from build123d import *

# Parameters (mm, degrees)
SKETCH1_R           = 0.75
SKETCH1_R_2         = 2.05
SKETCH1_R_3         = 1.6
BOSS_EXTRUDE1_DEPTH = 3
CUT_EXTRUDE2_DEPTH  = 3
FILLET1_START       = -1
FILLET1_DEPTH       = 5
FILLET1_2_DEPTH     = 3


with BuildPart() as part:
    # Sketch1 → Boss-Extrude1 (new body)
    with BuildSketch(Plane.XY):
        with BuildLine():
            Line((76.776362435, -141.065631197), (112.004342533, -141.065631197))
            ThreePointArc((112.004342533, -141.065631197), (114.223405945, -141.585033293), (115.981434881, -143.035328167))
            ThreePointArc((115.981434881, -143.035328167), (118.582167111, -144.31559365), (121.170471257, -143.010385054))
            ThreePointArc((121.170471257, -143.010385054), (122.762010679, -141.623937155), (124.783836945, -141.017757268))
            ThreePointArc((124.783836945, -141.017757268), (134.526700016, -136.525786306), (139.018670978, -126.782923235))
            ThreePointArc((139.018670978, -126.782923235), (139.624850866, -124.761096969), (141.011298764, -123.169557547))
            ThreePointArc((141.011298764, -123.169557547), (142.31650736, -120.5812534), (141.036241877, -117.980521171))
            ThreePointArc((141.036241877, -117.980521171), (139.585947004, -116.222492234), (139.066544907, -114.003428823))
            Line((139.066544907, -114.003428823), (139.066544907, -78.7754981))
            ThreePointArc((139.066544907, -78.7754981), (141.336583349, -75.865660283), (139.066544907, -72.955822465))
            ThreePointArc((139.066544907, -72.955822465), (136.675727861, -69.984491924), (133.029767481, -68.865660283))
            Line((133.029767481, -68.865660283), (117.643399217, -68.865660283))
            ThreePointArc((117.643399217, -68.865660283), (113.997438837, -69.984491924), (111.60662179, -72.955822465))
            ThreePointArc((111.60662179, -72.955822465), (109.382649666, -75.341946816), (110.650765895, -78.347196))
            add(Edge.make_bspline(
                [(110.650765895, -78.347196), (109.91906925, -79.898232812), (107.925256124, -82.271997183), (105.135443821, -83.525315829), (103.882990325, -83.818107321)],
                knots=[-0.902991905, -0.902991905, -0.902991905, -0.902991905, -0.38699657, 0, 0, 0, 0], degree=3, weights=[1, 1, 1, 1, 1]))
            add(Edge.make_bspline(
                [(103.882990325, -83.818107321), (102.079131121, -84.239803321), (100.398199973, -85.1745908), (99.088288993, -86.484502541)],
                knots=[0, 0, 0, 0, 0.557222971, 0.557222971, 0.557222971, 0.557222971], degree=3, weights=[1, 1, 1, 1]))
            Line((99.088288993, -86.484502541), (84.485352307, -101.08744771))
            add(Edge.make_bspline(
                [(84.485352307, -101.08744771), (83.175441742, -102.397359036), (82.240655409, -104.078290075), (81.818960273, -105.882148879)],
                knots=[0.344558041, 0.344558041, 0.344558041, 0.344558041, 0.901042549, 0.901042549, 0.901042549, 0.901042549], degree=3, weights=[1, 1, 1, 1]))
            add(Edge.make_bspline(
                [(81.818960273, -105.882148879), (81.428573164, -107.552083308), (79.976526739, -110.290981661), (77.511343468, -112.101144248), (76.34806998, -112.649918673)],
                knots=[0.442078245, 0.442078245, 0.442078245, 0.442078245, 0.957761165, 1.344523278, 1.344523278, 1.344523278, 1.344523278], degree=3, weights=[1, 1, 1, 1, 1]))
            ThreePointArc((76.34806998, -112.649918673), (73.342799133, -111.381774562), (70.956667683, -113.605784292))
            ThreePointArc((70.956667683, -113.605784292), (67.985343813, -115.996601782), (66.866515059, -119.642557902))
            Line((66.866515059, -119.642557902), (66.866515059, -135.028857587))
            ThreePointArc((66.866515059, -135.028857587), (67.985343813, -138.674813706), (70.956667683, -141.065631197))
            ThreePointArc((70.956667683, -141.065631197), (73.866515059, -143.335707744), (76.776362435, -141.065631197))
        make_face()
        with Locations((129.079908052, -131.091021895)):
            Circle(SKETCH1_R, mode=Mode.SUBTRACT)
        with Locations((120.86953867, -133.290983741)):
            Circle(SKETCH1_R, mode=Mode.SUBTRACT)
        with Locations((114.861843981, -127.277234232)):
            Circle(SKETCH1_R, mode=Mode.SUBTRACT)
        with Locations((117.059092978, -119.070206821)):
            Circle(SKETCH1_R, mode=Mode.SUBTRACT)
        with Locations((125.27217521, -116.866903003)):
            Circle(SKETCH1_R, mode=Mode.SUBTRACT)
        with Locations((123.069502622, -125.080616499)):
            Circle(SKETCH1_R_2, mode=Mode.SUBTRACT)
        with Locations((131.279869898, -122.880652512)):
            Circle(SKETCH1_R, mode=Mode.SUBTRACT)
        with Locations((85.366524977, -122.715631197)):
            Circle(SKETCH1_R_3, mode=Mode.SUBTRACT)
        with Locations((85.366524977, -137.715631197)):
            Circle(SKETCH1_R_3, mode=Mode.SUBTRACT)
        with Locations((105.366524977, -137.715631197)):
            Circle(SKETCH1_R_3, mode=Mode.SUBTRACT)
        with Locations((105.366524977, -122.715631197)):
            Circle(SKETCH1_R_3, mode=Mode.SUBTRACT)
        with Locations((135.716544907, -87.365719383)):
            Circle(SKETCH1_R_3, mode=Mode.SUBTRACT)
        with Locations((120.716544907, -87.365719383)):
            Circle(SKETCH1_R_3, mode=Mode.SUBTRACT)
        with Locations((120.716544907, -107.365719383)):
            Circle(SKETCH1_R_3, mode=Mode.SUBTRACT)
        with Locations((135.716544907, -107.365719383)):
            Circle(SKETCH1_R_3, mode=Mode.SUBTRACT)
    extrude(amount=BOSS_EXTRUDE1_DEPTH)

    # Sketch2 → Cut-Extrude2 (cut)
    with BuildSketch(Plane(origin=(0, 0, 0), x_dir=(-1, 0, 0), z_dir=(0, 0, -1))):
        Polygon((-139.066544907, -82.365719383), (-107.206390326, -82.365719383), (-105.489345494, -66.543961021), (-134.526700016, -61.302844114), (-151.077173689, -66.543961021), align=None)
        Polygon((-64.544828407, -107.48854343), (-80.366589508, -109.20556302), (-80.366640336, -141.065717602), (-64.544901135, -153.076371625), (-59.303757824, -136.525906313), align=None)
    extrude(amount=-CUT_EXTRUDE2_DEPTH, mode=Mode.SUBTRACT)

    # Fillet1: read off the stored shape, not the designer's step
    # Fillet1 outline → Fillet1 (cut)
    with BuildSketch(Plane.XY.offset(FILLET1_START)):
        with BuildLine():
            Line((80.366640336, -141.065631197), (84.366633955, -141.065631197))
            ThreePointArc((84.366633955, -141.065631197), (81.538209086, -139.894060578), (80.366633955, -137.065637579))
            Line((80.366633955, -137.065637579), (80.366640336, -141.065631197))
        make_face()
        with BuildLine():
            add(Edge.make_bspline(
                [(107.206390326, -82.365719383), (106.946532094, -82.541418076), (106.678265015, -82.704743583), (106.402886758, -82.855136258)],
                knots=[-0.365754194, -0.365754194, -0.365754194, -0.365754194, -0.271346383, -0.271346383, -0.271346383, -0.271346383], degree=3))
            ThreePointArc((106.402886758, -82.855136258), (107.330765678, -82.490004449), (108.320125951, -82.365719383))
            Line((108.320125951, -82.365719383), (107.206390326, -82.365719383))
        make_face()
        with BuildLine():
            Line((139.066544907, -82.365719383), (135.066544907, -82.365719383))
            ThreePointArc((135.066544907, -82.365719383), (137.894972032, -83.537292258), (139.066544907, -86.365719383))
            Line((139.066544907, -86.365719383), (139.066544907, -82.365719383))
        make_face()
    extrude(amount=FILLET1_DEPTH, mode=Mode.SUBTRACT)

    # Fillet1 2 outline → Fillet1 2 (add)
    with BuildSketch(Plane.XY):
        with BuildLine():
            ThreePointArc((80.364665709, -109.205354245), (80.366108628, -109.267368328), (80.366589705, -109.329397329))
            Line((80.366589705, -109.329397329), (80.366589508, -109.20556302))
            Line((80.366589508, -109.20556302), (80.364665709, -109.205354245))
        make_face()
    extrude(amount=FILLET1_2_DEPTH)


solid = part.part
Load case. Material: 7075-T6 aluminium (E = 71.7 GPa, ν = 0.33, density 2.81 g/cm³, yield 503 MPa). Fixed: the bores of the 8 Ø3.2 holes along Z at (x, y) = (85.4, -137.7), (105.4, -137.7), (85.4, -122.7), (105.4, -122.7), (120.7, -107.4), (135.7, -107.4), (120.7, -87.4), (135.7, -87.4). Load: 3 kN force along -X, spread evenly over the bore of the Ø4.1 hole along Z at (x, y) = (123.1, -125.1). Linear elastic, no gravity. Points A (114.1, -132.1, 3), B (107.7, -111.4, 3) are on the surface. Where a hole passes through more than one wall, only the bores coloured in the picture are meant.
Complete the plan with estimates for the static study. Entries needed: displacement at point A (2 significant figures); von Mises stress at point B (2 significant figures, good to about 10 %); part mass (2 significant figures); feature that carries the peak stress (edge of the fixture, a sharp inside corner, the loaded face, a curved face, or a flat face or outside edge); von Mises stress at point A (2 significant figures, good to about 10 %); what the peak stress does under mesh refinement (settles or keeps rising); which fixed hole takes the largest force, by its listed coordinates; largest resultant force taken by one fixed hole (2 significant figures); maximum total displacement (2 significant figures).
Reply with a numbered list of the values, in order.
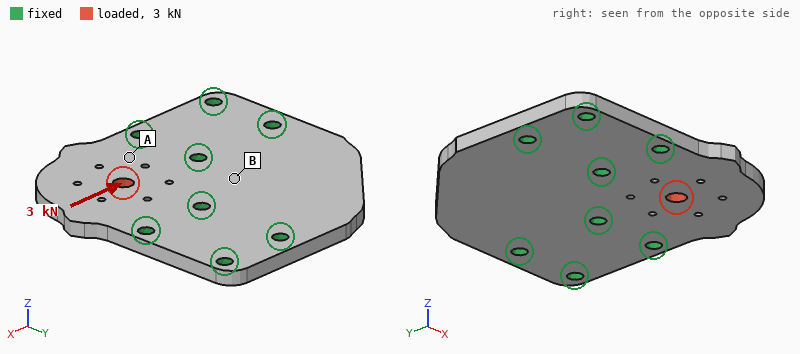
1. 4.4 µm
2. 8.8 MPa
3. 26 g
4. a sharp inside corner
5. 32 MPa
6. keeps rising
7. (105.4, -122.7)
8. 1.1 kN
9. 14 µm
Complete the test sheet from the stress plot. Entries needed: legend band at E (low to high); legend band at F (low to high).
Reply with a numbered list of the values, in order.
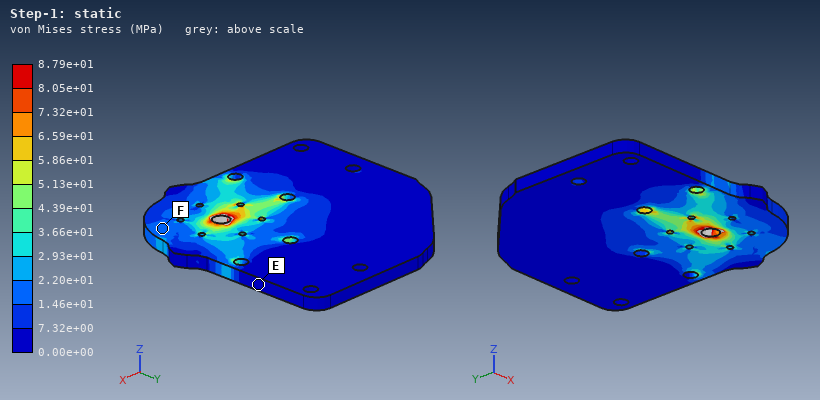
1. 0.00e+00 to 7.32e+00 MPa
2. 1.46e+01 to 2.20e+01 MPa
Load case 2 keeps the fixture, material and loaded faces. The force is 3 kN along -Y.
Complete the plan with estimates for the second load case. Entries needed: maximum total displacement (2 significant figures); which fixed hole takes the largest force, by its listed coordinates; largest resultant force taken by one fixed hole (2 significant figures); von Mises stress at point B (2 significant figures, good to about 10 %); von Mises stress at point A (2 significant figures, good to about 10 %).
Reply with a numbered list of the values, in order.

1. 14 µm
2. (120.7, -107.4)
3. 1.1 kN
4. 8.4 MPa
5. 29 MPa
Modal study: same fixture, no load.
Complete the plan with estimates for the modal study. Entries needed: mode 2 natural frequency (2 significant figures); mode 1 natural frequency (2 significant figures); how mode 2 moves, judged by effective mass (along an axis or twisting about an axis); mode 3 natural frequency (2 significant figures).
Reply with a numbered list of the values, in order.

1. 5500 Hz
2. 5200 Hz
3. along Z
4. 13 kHz
